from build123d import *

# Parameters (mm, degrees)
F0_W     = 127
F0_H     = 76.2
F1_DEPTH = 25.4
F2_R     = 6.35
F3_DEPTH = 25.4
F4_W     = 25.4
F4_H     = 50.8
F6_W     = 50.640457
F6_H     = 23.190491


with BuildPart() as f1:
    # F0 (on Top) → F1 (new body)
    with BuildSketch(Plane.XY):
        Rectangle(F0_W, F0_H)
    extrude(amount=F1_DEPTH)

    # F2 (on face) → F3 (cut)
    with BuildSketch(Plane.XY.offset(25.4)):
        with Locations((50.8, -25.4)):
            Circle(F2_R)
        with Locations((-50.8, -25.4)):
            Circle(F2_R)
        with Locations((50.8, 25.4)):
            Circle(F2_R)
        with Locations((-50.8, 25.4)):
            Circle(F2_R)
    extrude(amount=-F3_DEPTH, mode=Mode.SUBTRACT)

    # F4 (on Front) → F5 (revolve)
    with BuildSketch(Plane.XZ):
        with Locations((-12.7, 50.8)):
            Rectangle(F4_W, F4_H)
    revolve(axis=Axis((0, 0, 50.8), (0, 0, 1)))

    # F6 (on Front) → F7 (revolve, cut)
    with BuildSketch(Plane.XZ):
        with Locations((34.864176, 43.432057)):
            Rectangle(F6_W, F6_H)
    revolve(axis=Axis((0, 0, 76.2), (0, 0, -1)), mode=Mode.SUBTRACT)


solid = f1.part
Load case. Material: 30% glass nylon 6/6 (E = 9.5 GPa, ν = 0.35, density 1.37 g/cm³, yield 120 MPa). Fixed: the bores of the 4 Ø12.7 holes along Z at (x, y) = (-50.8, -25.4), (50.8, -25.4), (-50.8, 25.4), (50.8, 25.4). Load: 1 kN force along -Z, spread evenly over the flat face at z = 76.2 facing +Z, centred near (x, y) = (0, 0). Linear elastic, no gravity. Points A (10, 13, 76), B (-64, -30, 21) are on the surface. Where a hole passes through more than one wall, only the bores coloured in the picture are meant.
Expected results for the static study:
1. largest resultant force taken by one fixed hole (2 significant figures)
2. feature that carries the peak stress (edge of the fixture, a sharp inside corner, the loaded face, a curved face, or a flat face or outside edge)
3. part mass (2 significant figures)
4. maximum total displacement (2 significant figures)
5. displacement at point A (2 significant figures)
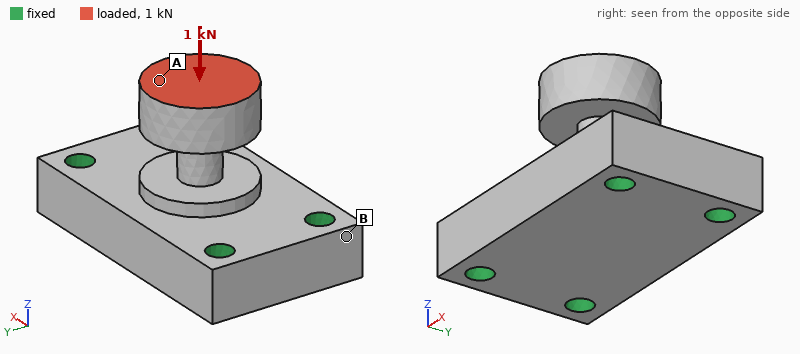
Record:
260 N
a curved face
400 g
22 µm
21 µm
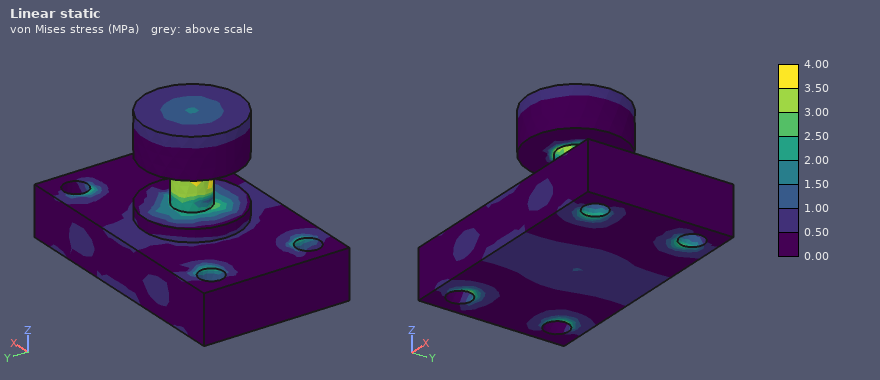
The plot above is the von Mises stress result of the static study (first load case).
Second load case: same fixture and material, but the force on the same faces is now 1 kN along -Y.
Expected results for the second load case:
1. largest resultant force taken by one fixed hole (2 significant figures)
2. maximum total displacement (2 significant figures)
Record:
650 N
0.77 mm
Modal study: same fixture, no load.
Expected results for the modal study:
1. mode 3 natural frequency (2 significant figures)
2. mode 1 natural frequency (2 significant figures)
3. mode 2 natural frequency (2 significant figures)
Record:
1500 Hz
1000 Hz
1000 Hz
